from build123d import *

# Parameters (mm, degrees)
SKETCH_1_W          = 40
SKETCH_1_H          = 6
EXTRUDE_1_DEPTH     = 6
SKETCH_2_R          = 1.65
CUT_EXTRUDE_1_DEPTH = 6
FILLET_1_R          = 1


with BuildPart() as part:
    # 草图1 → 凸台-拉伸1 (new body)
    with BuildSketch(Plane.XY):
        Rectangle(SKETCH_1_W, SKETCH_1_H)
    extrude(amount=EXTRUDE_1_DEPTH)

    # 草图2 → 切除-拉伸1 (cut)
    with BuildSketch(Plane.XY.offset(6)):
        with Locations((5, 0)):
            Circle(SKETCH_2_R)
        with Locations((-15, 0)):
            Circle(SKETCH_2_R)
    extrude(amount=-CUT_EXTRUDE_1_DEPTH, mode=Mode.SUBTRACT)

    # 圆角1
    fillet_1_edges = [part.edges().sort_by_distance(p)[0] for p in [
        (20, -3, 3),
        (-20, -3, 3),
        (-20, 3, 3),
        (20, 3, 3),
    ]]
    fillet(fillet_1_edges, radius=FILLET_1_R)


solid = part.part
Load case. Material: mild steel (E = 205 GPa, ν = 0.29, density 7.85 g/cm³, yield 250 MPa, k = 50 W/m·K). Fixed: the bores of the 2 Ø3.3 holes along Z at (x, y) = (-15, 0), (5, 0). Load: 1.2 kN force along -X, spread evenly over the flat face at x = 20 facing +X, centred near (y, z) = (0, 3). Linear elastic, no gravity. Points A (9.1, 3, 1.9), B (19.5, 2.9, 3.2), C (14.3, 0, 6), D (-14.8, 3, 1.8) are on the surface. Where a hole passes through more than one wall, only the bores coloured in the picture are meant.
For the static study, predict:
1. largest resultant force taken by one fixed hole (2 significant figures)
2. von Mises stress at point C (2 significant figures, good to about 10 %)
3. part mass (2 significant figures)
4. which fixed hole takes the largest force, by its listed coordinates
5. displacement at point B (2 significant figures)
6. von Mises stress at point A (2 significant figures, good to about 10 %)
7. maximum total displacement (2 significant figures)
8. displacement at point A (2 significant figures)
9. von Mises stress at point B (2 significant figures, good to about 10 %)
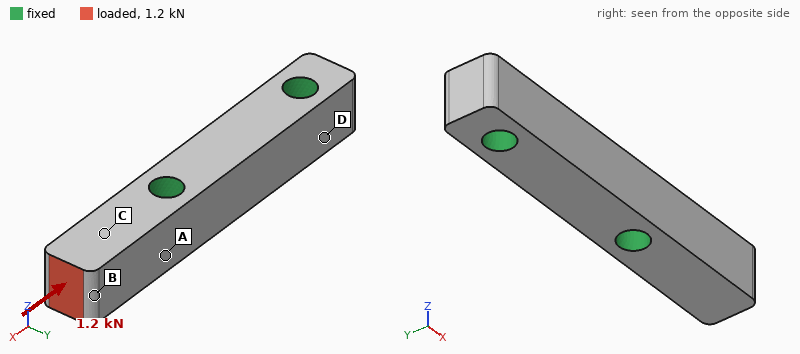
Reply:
1.2 kN
35 MPa
10 g
(5, 0)
1.9 µm
29 MPa
2.6 µm
0.56 µm
8.2 MPa
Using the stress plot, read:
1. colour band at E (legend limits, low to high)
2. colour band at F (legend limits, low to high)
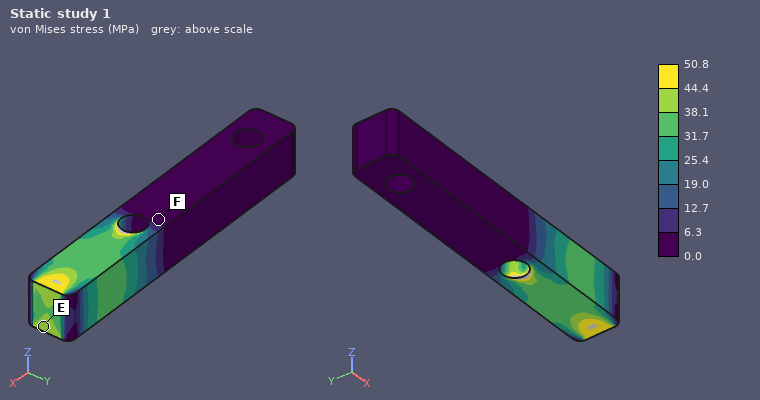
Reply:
38.1 to 44.4 MPa
0.0 to 6.3 MPa
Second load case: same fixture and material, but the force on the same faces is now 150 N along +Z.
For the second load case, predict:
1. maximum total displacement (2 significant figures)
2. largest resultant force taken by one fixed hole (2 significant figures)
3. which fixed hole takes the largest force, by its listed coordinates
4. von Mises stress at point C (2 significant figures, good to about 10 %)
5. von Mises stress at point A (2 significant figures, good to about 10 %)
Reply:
7.5 µm
150 N
(5, 0)
24 MPa
16 MPa
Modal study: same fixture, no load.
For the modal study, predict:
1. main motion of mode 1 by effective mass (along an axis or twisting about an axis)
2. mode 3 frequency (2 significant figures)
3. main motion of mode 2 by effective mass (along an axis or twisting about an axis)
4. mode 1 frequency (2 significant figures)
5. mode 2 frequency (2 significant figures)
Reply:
along Y
53 kHz
along Z
20 kHz
23 kHz
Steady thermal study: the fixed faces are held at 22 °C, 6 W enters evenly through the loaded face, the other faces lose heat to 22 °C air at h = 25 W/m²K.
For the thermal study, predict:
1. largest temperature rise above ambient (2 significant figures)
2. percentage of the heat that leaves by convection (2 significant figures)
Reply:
47 K
3.2 %
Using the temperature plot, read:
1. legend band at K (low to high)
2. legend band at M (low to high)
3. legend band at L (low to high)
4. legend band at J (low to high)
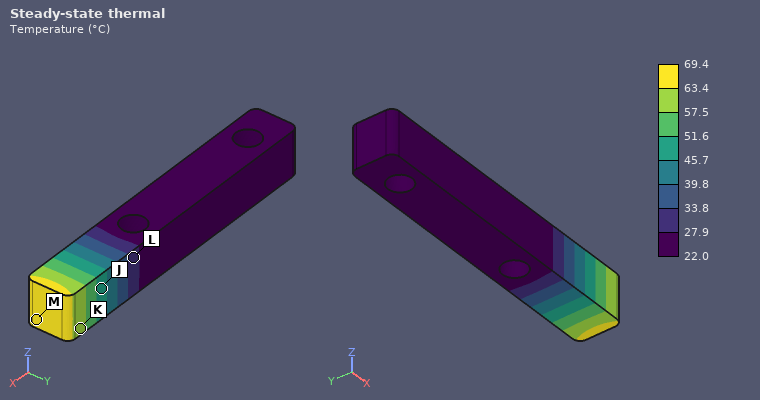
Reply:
57.5 to 63.4 °C
63.4 to 69.4 °C
27.9 to 33.8 °C
45.7 to 51.6 °C
